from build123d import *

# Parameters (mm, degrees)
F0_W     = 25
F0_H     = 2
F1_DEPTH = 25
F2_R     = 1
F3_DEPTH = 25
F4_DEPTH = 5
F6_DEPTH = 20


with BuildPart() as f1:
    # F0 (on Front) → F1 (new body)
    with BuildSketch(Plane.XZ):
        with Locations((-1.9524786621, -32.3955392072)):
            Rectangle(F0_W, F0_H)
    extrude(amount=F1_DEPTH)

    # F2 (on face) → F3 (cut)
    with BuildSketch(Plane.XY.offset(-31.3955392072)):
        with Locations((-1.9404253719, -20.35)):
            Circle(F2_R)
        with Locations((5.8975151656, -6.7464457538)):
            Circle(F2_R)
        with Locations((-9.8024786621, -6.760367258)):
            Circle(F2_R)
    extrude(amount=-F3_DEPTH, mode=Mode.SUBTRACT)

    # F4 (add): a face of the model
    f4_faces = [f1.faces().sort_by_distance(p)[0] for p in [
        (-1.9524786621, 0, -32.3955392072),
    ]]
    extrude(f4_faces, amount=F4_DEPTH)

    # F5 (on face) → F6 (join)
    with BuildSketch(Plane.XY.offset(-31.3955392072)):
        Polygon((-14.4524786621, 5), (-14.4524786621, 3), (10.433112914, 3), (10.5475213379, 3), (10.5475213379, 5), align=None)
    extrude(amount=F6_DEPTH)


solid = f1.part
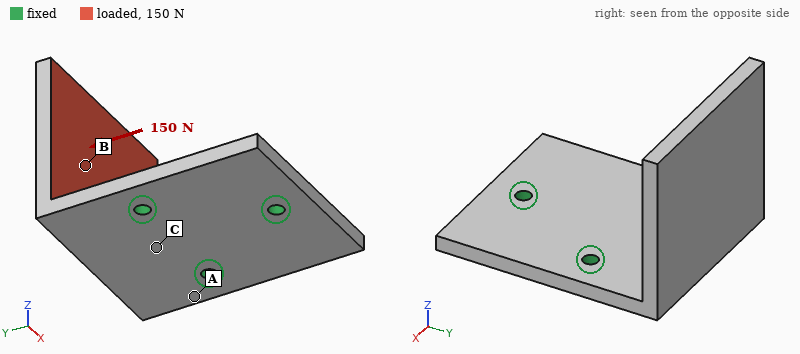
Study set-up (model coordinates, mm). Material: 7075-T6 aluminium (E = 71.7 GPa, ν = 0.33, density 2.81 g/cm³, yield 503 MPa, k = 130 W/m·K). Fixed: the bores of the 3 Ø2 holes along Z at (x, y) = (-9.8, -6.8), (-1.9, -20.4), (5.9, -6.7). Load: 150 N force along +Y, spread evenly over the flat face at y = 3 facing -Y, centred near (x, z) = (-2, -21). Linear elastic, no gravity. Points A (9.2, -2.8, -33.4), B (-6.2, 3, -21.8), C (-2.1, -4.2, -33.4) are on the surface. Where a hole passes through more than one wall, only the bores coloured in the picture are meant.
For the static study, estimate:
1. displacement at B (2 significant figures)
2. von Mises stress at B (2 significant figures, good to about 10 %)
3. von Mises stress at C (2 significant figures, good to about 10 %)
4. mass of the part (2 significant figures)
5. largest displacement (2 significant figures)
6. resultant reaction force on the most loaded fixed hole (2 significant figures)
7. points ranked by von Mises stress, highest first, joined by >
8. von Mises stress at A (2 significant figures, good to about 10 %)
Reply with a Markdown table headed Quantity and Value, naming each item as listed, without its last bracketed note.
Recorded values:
| Quantity | Value |
|---|---|
| displacement at B | 0.20 mm |
| von Mises stress at B | 23 MPa |
| von Mises stress at C | 68 MPa |
| mass of the part | 7.0 g |
| largest displacement | 0.43 mm |
| resultant reaction force on the most loaded fixed hole | 69 N |
| points ranked by von Mises stress, highest first, joined by > | A > C > B |
| von Mises stress at A | 98 MPa |
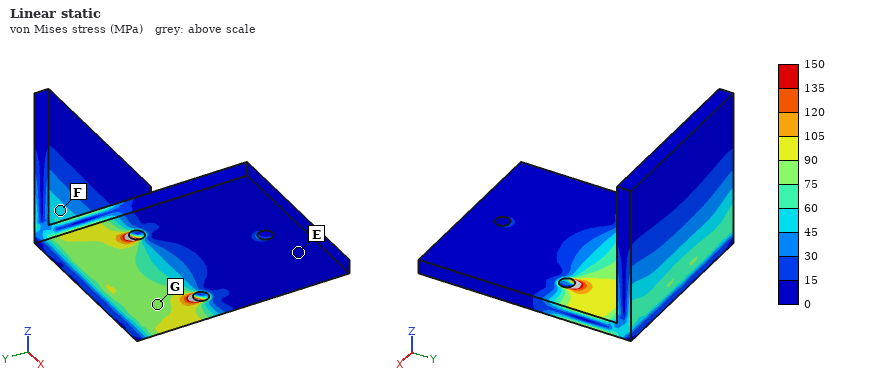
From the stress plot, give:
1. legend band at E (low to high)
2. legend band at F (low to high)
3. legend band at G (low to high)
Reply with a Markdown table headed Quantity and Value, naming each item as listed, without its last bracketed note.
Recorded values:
| Quantity | Value |
|---|---|
| legend band at E | 0 to 15 MPa |
| legend band at F | 45 to 60 MPa |
| legend band at G | 75 to 90 MPa |
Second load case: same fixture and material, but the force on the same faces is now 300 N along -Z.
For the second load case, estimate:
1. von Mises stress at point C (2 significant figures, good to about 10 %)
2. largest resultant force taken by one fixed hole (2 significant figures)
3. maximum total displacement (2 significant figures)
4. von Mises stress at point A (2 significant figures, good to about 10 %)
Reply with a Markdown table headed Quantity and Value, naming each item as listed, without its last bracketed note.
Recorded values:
| Quantity | Value |
|---|---|
| von Mises stress at point C | 82 MPa |
| largest resultant force taken by one fixed hole | 170 N |
| maximum total displacement | 0.24 mm |
| von Mises stress at point A | 110 MPa |
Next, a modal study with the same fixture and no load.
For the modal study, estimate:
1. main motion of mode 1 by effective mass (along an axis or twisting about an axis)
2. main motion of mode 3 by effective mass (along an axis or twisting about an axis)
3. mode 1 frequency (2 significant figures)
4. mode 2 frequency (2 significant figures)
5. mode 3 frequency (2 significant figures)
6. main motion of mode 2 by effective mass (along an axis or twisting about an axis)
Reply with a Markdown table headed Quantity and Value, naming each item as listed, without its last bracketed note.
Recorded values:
| Quantity | Value |
|---|---|
| main motion of mode 1 by effective mass | along Y |
| main motion of mode 3 by effective mass | along Z |
| mode 1 frequency | 2100 Hz |
| mode 2 frequency | 4200 Hz |
| mode 3 frequency | 6800 Hz |
| main motion of mode 2 by effective mass | along X |
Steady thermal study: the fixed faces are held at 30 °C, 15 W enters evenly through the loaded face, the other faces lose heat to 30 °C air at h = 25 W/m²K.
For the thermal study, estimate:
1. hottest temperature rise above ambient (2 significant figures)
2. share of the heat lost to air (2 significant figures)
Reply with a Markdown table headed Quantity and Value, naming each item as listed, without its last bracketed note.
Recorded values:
| Quantity | Value |
|---|---|
| hottest temperature rise above ambient | 48 K |
| share of the heat lost to air | 6.3 % |
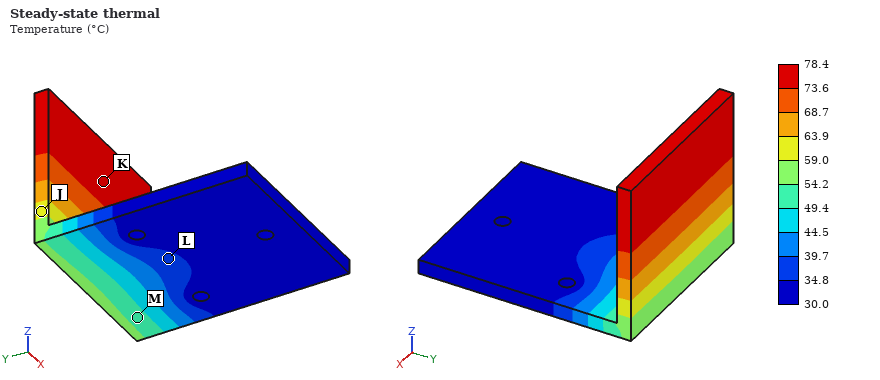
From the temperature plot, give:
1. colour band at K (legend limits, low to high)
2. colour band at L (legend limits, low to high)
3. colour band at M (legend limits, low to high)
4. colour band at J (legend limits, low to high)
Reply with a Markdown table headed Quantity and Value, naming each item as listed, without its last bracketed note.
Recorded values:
| Quantity | Value |
|---|---|
| colour band at K | 73.6 to 78.4 °C |
| colour band at L | 34.8 to 39.7 °C |
| colour band at M | 49.4 to 54.2 °C |
| colour band at J | 59.0 to 63.9 °C |
